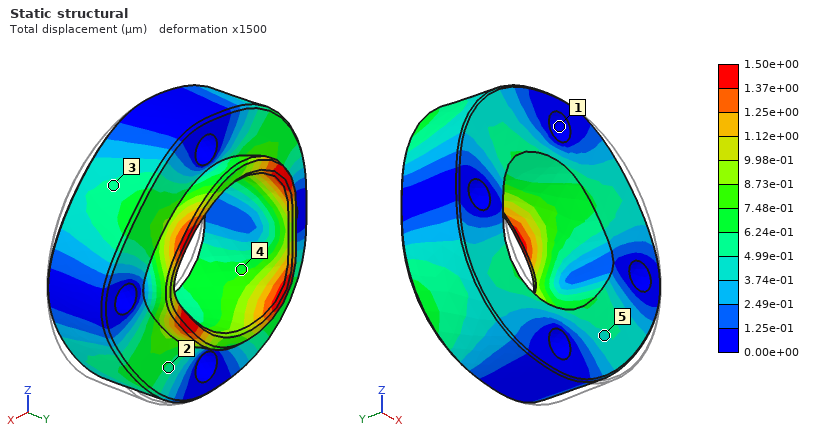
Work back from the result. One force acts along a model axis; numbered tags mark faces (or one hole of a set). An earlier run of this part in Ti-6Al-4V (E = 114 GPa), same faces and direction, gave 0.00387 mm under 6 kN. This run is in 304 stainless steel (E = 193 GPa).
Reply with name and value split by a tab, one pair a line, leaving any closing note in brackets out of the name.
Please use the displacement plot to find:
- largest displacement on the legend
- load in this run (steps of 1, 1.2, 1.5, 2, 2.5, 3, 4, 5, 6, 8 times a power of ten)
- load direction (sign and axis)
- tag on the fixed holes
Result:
largest displacement on the legend	1.50e+00 µm
load in this run	4 kN
load direction	-X
tag on the fixed holes	1
